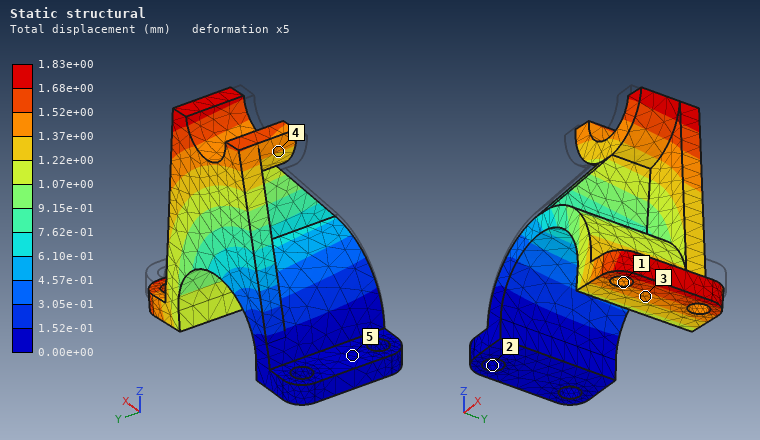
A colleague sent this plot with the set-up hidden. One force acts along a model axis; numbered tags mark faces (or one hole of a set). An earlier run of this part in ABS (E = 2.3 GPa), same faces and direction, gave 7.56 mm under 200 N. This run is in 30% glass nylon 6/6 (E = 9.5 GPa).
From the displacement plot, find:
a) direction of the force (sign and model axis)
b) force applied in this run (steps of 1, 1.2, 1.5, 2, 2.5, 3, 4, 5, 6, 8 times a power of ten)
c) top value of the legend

-Z
200 N
1.83e+00 mm
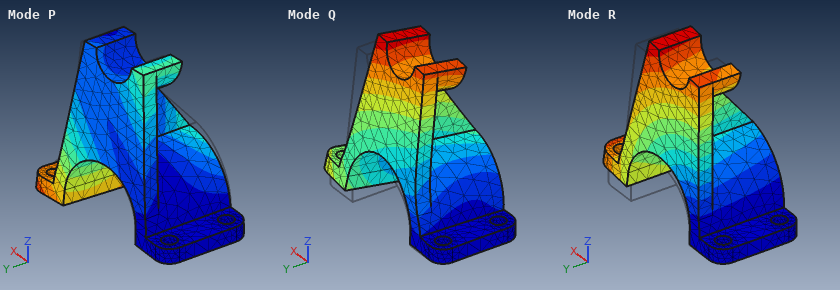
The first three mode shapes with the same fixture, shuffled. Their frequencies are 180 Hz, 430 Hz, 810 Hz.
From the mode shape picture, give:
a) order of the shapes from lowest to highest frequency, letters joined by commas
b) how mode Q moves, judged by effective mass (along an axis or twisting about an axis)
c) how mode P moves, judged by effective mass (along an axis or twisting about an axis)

R, P, Q
along Y
along Y
